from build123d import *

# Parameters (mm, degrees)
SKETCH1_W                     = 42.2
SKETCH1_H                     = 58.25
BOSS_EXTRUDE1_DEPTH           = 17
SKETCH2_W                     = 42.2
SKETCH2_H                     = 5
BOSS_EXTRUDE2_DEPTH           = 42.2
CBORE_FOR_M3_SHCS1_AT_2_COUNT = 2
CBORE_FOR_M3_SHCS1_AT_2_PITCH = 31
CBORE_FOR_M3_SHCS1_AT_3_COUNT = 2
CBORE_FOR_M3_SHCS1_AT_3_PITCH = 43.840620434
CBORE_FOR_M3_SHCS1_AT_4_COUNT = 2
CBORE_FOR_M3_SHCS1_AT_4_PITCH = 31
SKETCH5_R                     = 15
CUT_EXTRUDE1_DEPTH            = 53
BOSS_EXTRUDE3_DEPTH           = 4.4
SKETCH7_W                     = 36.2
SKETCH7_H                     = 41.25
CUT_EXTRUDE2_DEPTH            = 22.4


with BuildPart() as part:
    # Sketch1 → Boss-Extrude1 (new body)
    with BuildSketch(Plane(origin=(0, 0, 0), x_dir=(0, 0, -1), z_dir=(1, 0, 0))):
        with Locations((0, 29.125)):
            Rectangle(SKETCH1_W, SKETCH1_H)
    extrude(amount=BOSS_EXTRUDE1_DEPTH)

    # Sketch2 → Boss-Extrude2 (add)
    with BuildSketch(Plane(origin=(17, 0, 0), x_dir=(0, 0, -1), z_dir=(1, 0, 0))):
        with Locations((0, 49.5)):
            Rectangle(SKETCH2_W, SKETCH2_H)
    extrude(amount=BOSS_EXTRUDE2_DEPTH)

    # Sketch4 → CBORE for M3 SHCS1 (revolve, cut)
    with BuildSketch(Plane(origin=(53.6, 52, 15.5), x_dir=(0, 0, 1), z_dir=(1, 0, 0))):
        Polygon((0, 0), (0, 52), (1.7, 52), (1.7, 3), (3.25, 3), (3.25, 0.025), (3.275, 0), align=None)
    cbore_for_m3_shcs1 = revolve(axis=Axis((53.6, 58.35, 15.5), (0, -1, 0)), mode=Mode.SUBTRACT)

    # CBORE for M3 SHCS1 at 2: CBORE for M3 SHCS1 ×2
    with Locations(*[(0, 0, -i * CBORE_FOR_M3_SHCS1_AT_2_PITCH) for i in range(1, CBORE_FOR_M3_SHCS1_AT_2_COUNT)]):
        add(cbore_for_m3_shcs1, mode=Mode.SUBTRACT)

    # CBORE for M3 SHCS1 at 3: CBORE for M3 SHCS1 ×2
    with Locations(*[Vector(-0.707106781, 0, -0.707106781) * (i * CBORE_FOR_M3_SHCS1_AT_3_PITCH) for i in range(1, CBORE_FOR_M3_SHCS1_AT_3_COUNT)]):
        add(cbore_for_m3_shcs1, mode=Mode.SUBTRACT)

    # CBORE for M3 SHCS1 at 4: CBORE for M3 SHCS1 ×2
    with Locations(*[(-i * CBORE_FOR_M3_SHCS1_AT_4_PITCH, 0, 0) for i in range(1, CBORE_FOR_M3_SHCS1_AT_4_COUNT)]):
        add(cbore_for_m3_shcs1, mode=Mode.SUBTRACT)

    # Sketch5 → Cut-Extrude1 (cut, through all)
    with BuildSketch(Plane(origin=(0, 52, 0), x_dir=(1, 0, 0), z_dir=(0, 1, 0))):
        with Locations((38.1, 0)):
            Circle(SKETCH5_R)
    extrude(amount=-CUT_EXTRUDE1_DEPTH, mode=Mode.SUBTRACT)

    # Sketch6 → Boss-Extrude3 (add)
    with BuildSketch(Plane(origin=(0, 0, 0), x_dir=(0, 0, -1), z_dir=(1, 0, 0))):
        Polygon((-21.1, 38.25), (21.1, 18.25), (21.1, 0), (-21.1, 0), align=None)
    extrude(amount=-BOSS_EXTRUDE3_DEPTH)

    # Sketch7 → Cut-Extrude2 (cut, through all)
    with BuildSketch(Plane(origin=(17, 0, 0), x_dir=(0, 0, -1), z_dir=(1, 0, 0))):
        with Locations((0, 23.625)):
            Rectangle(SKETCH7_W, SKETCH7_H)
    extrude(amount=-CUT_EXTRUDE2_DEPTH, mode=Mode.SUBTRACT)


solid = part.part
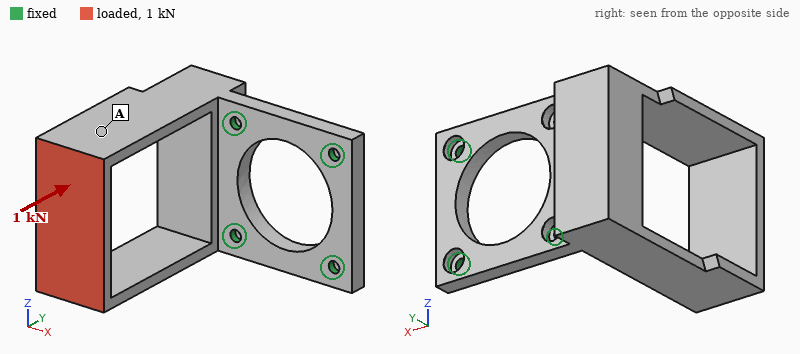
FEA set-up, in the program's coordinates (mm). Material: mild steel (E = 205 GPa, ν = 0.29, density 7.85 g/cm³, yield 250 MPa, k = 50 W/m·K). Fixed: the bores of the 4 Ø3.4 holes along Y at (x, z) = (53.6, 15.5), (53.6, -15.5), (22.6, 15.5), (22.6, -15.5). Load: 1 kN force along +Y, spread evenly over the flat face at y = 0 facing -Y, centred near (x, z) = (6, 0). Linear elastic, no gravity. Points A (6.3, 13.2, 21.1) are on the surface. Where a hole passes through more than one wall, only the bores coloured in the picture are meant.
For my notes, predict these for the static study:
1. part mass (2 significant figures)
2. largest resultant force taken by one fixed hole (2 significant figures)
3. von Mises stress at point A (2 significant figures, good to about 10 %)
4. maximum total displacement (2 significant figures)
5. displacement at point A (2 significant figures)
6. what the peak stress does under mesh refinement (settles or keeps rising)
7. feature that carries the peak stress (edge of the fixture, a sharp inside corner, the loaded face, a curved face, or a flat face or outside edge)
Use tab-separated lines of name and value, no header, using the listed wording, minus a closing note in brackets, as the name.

part mass	180 g
largest resultant force taken by one fixed hole	790 N
von Mises stress at point A	29 MPa
maximum total displacement	0.20 mm
displacement at point A	0.12 mm
what the peak stress does under mesh refinement	keeps rising
feature that carries the peak stress	edge of the fixture
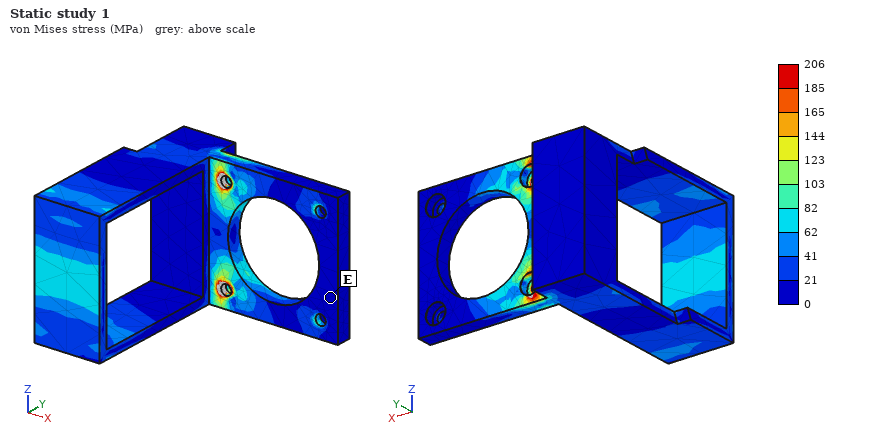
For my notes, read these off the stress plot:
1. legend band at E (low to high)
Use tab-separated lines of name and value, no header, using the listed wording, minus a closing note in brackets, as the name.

legend band at E	0 to 21 MPa
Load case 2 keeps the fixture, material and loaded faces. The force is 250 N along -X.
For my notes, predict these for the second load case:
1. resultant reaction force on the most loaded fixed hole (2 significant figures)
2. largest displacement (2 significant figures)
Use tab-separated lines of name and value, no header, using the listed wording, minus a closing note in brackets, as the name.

resultant reaction force on the most loaded fixed hole	480 N
largest displacement	0.17 mm
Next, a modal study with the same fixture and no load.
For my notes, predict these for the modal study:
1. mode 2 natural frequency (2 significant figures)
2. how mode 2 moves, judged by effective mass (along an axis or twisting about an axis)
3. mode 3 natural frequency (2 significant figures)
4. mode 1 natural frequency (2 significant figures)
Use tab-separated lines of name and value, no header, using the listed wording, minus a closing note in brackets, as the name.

mode 2 natural frequency	1100 Hz
how mode 2 moves, judged by effective mass	along Z
mode 3 natural frequency	3700 Hz
mode 1 natural frequency	1000 Hz
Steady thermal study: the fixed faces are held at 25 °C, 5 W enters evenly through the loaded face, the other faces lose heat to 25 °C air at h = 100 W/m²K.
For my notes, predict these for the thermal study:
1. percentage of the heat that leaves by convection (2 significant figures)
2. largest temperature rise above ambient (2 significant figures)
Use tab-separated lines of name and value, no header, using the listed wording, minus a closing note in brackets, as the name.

percentage of the heat that leaves by convection	89 %
largest temperature rise above ambient	17 K
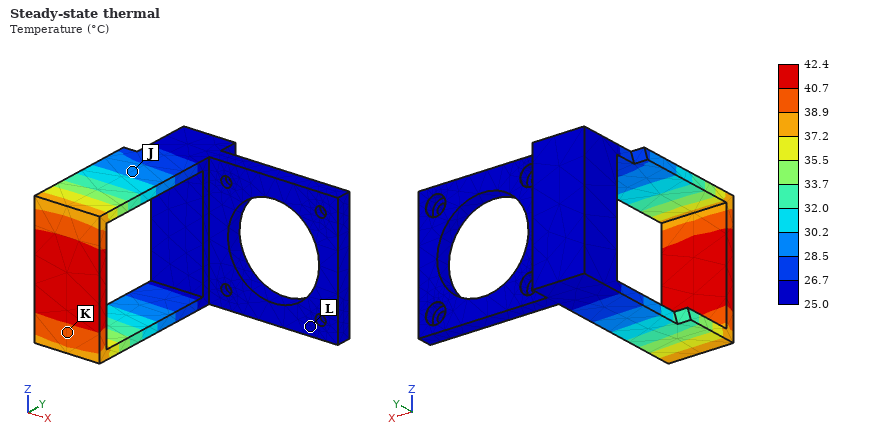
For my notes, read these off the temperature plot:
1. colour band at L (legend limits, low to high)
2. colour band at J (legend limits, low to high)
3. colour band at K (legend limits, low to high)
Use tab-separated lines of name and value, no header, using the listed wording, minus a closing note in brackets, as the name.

colour band at L	25.0 to 26.7 °C
colour band at J	28.5 to 30.2 °C
colour band at K	38.9 to 40.7 °C
